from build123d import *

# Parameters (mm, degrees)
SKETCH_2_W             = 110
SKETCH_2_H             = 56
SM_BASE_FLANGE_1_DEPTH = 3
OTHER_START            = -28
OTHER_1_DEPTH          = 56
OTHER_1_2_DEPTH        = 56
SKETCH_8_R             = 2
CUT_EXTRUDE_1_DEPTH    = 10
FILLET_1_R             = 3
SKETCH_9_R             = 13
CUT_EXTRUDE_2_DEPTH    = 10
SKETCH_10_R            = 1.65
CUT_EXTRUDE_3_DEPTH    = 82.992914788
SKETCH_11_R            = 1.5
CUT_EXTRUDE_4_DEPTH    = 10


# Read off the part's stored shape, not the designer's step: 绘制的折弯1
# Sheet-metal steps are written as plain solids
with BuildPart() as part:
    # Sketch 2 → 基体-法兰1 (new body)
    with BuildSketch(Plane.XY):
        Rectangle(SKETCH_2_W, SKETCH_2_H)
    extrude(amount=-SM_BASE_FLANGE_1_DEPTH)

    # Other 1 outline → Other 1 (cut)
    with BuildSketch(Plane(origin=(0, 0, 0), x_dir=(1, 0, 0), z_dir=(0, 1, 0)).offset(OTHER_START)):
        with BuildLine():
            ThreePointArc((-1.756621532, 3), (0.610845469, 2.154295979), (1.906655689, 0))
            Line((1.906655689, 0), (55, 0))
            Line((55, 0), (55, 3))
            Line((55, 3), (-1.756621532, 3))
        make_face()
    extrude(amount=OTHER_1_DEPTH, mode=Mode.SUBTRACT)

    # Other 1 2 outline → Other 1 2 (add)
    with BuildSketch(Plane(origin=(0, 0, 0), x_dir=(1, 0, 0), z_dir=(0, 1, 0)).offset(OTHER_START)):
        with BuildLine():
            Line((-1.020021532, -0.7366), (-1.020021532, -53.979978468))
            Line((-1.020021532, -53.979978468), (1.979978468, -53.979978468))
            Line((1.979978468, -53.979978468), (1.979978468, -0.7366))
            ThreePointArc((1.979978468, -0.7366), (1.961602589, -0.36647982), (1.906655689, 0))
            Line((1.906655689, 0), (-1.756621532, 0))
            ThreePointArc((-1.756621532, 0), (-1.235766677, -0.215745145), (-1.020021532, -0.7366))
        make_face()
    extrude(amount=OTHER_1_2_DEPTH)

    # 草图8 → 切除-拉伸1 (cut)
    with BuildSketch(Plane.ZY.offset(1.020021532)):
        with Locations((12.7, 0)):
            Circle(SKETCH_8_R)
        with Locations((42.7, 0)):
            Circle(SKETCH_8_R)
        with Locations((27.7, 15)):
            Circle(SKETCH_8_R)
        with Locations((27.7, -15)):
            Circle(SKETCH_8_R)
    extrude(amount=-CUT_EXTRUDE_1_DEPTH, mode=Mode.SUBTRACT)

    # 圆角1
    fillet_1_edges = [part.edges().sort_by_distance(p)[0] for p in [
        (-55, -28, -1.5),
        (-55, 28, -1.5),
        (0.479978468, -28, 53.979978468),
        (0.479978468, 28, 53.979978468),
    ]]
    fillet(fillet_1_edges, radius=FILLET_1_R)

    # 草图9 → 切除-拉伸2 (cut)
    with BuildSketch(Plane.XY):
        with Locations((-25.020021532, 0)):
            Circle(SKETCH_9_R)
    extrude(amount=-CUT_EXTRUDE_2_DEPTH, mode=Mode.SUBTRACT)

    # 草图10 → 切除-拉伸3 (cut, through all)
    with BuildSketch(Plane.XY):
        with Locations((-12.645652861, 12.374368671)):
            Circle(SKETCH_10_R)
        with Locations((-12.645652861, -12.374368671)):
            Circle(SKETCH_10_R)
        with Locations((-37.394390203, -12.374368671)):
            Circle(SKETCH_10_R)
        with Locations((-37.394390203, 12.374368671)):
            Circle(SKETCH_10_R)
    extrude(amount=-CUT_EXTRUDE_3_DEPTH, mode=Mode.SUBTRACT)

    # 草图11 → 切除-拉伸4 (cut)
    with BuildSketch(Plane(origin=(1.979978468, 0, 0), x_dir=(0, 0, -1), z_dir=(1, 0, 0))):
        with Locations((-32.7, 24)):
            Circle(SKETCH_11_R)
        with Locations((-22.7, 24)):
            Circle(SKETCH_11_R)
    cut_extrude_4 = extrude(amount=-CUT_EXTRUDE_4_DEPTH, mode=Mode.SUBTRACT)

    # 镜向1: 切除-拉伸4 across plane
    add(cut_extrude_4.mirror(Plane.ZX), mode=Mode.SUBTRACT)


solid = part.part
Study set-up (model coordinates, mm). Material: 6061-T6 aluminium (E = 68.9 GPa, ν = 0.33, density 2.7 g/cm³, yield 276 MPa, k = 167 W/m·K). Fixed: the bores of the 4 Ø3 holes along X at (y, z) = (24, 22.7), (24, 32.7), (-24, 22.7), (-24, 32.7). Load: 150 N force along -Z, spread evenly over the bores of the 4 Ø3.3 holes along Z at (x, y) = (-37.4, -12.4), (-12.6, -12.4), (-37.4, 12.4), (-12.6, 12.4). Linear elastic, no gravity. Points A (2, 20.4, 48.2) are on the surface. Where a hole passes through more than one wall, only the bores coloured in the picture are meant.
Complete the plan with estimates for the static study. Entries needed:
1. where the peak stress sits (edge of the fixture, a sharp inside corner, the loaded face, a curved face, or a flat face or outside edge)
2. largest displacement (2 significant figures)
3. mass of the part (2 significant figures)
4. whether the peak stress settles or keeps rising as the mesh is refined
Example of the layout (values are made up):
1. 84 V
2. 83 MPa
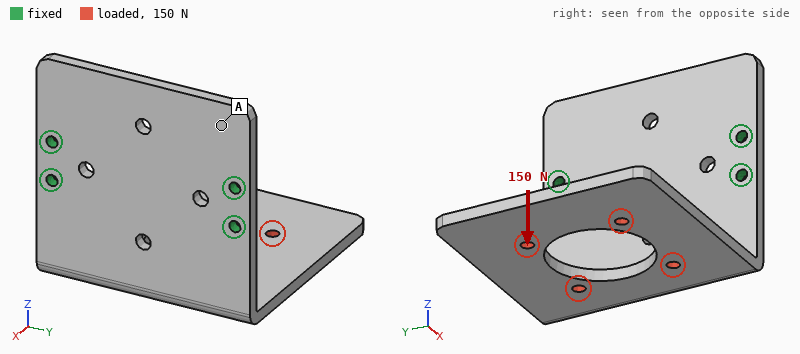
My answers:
1. edge of the fixture
2. 1.0 mm
3. 45 g
4. keeps rising
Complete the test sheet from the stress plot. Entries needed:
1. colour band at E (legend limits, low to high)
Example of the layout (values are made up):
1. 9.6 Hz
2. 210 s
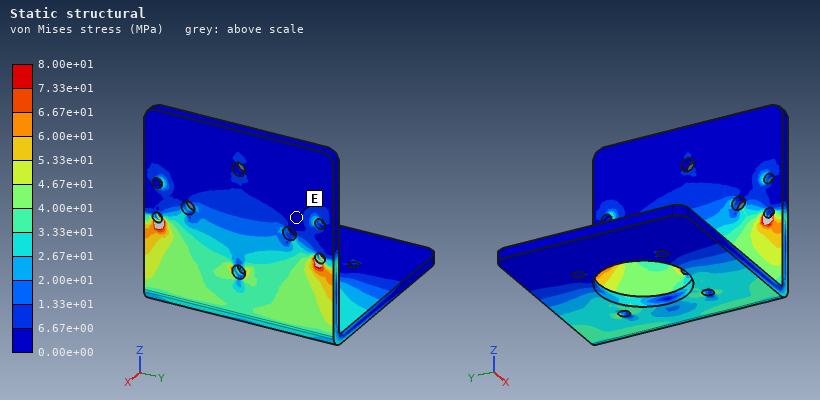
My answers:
1. 0.00e+00 to 6.67e+00 MPa
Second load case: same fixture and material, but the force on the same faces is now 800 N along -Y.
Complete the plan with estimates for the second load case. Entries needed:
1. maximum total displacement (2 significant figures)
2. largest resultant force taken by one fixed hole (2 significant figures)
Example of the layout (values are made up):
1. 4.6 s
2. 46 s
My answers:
1. 0.90 mm
2. 720 N
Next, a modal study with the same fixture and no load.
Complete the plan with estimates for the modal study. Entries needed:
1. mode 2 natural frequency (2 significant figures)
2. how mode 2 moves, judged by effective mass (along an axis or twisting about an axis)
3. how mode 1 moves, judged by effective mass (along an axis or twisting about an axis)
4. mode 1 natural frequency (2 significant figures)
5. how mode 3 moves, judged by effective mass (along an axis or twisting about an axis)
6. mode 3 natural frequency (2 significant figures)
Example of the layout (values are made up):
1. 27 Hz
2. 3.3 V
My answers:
1. 1100 Hz
2. along Y
3. along Z
4. 460 Hz
5. along X
6. 1600 Hz
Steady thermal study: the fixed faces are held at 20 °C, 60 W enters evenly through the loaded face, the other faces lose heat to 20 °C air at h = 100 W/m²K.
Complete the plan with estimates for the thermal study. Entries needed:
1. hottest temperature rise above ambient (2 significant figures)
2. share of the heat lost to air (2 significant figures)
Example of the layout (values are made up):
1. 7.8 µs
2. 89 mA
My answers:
1. 70 K
2. 60 %
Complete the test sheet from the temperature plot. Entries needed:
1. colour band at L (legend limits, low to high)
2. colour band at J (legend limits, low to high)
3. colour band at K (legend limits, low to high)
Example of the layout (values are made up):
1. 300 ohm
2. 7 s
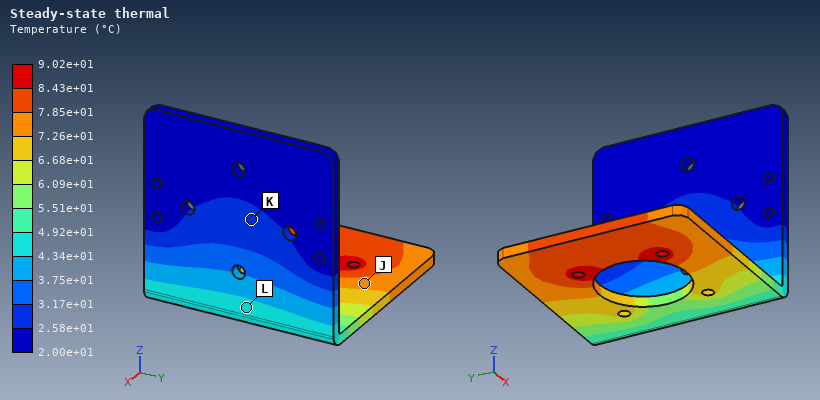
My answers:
1. 4.34e+01 to 4.92e+01 °C
2. 7.26e+01 to 7.85e+01 °C
3. 2.58e+01 to 3.17e+01 °C
